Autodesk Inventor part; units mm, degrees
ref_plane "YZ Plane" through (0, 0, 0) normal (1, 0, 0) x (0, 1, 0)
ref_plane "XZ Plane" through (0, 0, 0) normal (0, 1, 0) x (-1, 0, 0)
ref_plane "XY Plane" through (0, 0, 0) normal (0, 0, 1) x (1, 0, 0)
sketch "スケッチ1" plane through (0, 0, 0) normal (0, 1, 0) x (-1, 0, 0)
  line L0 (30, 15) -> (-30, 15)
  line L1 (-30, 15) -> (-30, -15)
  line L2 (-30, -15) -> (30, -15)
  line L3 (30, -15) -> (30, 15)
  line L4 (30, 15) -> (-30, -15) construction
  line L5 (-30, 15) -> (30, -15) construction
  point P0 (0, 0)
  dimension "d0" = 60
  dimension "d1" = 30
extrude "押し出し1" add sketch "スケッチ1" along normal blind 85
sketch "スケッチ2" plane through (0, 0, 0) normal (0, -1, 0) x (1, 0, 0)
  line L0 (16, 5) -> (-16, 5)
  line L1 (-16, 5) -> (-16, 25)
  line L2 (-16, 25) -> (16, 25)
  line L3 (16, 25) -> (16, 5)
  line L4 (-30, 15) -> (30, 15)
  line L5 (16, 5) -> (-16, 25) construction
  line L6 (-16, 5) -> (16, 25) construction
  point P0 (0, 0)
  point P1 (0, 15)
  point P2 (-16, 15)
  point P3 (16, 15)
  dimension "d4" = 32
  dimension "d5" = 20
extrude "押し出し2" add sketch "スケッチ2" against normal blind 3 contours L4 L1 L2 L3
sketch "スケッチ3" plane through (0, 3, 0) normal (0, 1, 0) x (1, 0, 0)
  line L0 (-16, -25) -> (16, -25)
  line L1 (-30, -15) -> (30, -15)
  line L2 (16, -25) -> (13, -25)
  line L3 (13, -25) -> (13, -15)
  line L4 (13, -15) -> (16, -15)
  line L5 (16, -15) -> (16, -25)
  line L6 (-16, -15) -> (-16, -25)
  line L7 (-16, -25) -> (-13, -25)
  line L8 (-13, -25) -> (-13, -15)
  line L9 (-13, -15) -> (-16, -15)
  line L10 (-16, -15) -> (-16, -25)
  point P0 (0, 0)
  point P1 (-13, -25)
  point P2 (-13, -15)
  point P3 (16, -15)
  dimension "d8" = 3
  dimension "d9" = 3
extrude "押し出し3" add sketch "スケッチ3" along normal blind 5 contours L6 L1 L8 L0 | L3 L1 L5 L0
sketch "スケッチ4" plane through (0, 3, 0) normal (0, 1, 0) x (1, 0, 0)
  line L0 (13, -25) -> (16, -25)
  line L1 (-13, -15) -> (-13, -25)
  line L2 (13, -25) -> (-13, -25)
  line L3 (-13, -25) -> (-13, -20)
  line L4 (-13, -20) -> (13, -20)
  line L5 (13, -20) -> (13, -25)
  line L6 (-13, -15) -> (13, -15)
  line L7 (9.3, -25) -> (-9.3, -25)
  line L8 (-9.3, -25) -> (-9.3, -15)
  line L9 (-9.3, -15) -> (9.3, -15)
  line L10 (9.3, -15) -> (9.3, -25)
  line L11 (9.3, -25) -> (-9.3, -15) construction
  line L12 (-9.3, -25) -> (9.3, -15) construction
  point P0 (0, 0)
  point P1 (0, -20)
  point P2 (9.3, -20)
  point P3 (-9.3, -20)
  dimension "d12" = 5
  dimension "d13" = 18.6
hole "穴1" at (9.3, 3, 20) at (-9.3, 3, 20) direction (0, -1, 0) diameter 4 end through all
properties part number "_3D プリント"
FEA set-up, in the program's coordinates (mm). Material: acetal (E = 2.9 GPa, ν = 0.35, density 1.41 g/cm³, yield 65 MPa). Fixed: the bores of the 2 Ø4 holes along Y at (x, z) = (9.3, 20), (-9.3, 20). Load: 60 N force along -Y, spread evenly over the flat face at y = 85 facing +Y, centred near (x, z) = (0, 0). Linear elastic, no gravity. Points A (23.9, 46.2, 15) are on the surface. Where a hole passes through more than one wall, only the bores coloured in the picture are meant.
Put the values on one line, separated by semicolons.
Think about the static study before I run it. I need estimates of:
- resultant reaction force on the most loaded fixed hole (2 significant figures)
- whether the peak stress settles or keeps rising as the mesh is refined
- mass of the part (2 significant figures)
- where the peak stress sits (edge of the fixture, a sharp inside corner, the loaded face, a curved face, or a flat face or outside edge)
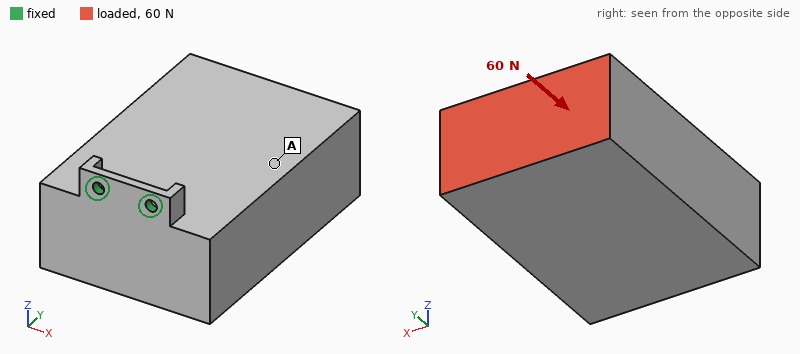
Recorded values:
31 N; keeps rising; 220 g; edge of the fixture
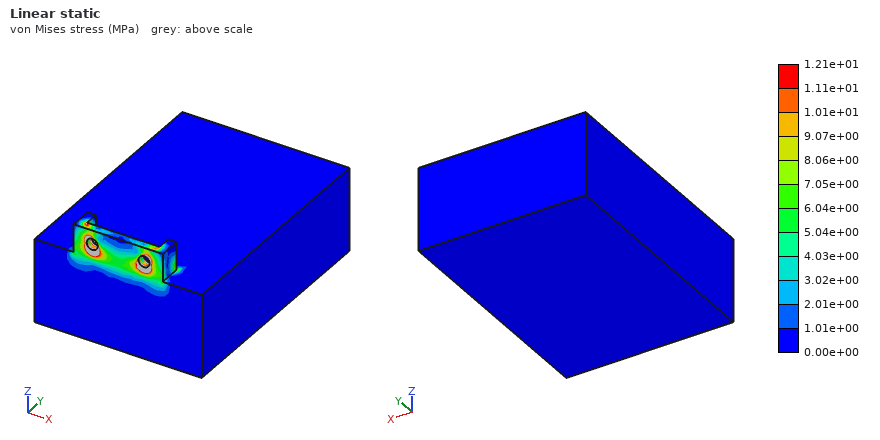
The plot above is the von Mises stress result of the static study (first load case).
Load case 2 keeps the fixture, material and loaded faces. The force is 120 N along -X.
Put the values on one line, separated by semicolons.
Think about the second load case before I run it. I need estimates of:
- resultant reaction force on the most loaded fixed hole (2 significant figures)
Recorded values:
460 N
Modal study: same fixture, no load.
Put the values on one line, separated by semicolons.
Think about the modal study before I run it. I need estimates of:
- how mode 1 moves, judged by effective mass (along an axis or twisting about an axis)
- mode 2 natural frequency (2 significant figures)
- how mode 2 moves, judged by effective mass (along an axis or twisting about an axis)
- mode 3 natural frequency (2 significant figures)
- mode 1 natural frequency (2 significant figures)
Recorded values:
along Z; 180 Hz; along X; 640 Hz; 57 Hz
